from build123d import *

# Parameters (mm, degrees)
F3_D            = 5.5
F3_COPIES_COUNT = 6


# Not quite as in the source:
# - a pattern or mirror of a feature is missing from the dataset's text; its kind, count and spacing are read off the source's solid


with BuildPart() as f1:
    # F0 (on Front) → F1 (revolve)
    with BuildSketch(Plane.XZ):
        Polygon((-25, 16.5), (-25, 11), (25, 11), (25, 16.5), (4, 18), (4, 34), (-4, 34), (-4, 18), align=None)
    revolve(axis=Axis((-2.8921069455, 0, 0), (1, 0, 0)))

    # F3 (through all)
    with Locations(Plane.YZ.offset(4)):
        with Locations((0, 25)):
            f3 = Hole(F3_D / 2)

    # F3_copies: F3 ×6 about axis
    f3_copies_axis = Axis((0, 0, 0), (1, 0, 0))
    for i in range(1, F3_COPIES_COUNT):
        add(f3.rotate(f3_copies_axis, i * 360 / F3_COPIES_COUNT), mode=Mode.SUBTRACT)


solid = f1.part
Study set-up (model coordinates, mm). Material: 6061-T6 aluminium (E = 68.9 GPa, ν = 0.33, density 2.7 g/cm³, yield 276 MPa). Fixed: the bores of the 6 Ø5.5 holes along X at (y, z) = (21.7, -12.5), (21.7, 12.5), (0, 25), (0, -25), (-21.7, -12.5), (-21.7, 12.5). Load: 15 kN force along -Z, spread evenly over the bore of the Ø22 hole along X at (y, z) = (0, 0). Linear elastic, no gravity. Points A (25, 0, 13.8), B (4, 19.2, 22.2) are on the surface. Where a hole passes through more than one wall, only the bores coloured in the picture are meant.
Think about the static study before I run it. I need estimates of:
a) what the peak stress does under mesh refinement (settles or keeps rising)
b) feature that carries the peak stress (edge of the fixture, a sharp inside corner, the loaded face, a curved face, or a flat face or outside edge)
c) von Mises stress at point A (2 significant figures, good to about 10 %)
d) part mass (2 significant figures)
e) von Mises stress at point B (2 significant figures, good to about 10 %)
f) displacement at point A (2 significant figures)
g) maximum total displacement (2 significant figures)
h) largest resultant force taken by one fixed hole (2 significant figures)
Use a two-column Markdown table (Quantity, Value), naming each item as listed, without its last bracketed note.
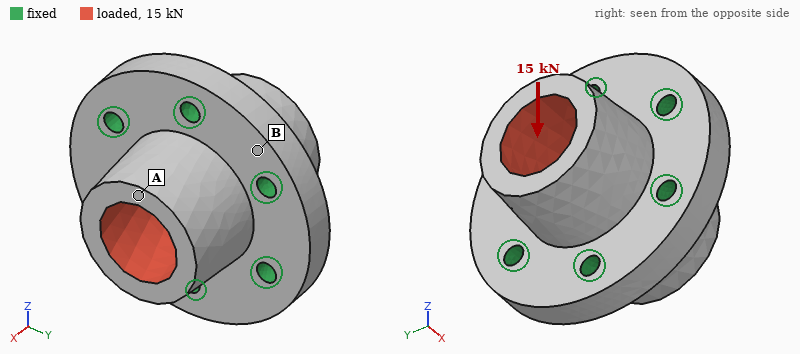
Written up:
| Quantity | Value |
|---|---|
| what the peak stress does under mesh refinement | keeps rising |
| feature that carries the peak stress | edge of the fixture |
| von Mises stress at point A | 15 MPa |
| part mass | 130 g |
| von Mises stress at point B | 7.6 MPa |
| displacement at point A | 15 µm |
| maximum total displacement | 16 µm |
| largest resultant force taken by one fixed hole | 3.4 kN |
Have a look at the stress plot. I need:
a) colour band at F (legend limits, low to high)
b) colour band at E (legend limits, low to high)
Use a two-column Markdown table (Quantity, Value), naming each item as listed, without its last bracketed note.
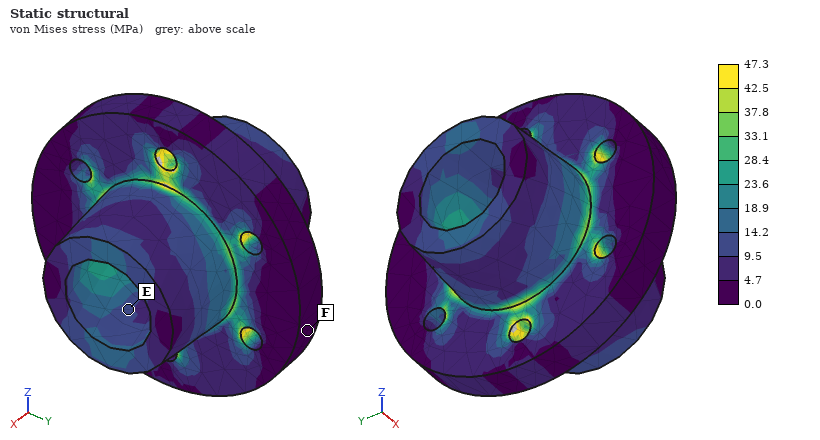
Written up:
| Quantity | Value |
|---|---|
| colour band at F | 0.0 to 4.7 MPa |
| colour band at E | 9.5 to 14.2 MPa |
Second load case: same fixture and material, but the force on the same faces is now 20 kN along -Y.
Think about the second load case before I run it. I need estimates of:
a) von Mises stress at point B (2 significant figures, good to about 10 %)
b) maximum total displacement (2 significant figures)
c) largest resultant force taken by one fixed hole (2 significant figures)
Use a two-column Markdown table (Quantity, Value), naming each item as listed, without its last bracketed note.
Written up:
| Quantity | Value |
|---|---|
| von Mises stress at point B | 6.1 MPa |
| maximum total displacement | 21 µm |
| largest resultant force taken by one fixed hole | 4.1 kN |
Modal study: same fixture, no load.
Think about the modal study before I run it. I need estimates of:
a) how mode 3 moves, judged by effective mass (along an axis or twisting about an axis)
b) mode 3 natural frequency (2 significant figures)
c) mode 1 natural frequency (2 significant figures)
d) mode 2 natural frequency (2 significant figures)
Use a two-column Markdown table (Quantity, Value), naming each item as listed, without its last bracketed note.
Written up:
| Quantity | Value |
|---|---|
| how mode 3 moves, judged by effective mass | along X |
| mode 3 natural frequency | 22 kHz |
| mode 1 natural frequency | 18 kHz |
| mode 2 natural frequency | 18 kHz |
